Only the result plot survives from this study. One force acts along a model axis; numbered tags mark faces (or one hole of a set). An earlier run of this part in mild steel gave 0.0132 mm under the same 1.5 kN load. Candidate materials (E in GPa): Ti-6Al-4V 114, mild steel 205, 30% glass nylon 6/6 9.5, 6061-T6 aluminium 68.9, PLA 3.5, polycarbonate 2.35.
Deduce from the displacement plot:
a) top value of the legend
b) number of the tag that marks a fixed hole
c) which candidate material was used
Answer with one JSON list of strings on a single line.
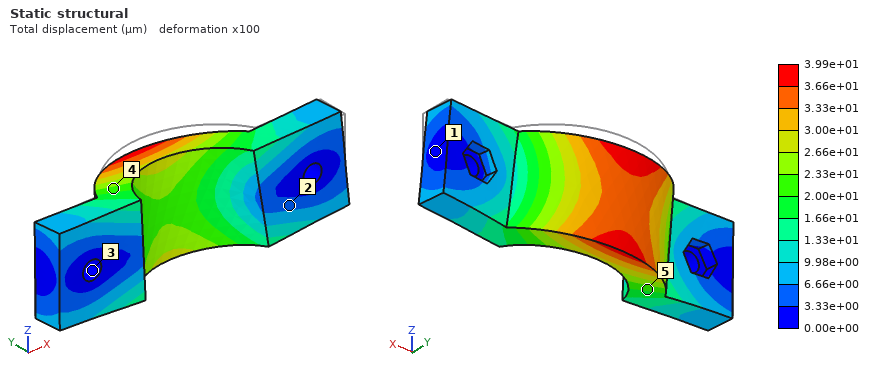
["3.99e+01 µm", "3", "6061-T6 aluminium"]
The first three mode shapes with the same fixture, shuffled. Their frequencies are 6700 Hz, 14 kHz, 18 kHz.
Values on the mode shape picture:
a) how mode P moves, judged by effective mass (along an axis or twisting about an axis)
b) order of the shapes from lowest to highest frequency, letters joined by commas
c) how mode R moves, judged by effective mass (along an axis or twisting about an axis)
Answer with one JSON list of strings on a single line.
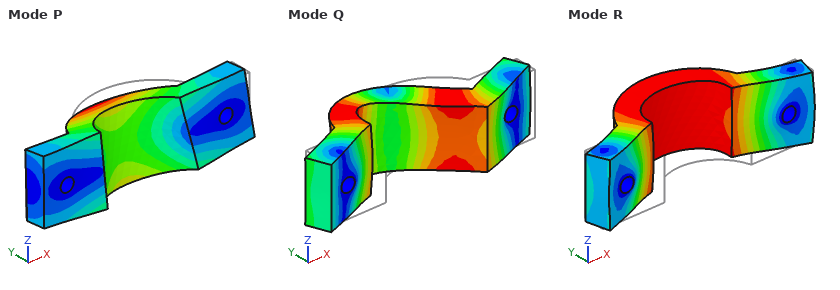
["along Z", "P, R, Q", "along Y"]
